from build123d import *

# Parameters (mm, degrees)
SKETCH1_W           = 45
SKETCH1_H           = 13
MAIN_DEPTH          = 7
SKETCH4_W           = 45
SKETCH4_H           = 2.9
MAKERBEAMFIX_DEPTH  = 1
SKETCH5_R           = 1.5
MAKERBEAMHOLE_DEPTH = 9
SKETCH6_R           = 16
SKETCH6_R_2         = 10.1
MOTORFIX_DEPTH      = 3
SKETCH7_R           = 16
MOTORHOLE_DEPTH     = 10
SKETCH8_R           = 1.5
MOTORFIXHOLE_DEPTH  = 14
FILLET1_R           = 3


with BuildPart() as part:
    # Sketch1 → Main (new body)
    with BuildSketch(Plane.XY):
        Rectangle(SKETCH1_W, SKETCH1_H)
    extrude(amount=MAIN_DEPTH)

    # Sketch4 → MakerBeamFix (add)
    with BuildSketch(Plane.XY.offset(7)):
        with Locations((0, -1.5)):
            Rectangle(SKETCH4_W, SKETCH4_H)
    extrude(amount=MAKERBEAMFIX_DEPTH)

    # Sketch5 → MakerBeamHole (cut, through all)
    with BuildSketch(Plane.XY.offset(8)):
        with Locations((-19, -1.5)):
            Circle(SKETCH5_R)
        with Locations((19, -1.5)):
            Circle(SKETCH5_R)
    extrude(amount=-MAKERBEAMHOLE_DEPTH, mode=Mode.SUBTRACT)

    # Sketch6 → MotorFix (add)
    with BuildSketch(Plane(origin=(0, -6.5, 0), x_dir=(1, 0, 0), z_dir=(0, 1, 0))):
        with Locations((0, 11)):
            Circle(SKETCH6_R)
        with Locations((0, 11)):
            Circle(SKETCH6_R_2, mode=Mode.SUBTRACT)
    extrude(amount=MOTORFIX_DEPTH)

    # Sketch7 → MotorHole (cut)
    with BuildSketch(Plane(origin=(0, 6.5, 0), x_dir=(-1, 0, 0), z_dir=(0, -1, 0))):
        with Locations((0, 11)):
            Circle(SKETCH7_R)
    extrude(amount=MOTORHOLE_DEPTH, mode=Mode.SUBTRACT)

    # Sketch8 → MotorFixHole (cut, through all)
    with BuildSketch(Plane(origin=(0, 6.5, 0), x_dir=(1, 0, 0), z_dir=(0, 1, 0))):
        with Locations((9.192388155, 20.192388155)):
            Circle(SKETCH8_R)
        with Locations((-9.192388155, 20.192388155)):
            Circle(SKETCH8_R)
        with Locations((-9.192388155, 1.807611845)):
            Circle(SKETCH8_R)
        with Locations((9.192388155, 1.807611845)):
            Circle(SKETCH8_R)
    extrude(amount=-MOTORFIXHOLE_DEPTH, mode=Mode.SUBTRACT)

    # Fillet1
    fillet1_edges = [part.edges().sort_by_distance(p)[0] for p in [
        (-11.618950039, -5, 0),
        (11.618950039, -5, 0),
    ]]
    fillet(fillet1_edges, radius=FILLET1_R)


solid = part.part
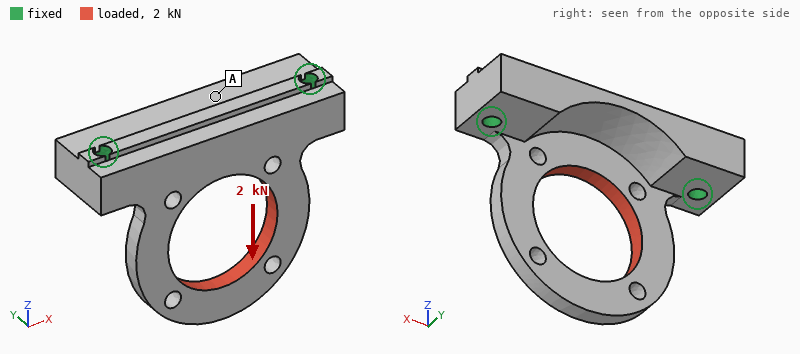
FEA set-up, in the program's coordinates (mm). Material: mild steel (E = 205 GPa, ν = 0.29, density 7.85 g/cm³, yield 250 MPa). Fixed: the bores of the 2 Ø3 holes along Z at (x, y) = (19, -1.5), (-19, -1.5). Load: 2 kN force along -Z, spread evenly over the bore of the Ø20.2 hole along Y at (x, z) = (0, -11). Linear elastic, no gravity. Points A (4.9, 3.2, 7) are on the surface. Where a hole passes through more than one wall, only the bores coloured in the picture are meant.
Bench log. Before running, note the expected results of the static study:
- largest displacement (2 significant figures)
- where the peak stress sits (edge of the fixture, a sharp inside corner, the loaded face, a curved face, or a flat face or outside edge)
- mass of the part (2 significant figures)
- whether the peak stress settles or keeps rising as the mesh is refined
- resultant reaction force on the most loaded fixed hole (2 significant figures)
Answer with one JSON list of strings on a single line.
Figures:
["18 µm", "edge of the fixture", "35 g", "keeps rising", "1.0 kN"]
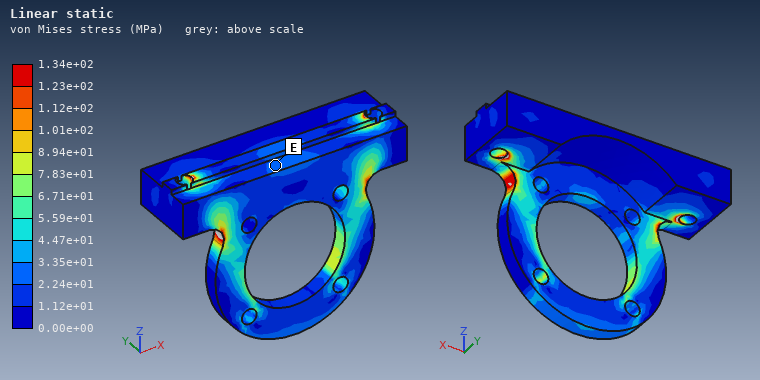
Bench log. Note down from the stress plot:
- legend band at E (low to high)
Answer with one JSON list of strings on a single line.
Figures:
["2.24e+01 to 3.35e+01 MPa"]
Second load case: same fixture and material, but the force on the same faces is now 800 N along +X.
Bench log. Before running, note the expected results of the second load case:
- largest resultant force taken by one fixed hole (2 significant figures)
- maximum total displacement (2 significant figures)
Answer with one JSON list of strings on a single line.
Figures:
["530 N", "21 µm"]
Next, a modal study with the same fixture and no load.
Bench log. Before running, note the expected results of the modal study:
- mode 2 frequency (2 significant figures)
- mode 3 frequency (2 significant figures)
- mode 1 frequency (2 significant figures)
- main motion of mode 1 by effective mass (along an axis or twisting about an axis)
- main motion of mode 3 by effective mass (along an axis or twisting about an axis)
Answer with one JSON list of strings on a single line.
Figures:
["6700 Hz", "10 kHz", "2600 Hz", "along Y", "along X"]
